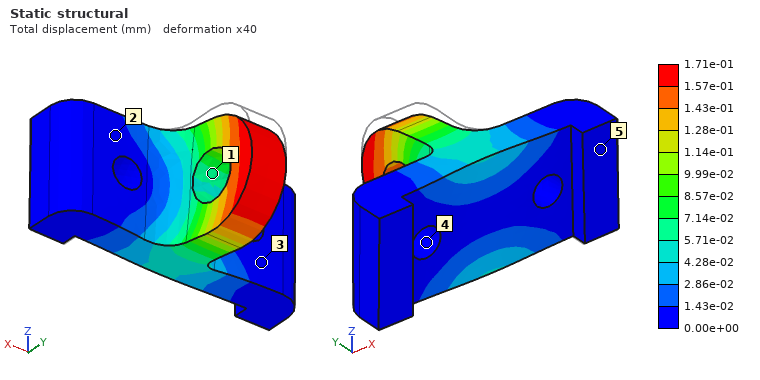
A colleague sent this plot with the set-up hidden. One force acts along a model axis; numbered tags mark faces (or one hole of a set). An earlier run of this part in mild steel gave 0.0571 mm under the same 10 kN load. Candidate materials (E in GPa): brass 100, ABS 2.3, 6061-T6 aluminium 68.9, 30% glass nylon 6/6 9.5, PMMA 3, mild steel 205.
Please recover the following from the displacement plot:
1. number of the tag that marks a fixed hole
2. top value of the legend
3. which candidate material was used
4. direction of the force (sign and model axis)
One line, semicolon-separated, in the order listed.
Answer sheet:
4; 1.71e-01 mm; 6061-T6 aluminium; -Z
